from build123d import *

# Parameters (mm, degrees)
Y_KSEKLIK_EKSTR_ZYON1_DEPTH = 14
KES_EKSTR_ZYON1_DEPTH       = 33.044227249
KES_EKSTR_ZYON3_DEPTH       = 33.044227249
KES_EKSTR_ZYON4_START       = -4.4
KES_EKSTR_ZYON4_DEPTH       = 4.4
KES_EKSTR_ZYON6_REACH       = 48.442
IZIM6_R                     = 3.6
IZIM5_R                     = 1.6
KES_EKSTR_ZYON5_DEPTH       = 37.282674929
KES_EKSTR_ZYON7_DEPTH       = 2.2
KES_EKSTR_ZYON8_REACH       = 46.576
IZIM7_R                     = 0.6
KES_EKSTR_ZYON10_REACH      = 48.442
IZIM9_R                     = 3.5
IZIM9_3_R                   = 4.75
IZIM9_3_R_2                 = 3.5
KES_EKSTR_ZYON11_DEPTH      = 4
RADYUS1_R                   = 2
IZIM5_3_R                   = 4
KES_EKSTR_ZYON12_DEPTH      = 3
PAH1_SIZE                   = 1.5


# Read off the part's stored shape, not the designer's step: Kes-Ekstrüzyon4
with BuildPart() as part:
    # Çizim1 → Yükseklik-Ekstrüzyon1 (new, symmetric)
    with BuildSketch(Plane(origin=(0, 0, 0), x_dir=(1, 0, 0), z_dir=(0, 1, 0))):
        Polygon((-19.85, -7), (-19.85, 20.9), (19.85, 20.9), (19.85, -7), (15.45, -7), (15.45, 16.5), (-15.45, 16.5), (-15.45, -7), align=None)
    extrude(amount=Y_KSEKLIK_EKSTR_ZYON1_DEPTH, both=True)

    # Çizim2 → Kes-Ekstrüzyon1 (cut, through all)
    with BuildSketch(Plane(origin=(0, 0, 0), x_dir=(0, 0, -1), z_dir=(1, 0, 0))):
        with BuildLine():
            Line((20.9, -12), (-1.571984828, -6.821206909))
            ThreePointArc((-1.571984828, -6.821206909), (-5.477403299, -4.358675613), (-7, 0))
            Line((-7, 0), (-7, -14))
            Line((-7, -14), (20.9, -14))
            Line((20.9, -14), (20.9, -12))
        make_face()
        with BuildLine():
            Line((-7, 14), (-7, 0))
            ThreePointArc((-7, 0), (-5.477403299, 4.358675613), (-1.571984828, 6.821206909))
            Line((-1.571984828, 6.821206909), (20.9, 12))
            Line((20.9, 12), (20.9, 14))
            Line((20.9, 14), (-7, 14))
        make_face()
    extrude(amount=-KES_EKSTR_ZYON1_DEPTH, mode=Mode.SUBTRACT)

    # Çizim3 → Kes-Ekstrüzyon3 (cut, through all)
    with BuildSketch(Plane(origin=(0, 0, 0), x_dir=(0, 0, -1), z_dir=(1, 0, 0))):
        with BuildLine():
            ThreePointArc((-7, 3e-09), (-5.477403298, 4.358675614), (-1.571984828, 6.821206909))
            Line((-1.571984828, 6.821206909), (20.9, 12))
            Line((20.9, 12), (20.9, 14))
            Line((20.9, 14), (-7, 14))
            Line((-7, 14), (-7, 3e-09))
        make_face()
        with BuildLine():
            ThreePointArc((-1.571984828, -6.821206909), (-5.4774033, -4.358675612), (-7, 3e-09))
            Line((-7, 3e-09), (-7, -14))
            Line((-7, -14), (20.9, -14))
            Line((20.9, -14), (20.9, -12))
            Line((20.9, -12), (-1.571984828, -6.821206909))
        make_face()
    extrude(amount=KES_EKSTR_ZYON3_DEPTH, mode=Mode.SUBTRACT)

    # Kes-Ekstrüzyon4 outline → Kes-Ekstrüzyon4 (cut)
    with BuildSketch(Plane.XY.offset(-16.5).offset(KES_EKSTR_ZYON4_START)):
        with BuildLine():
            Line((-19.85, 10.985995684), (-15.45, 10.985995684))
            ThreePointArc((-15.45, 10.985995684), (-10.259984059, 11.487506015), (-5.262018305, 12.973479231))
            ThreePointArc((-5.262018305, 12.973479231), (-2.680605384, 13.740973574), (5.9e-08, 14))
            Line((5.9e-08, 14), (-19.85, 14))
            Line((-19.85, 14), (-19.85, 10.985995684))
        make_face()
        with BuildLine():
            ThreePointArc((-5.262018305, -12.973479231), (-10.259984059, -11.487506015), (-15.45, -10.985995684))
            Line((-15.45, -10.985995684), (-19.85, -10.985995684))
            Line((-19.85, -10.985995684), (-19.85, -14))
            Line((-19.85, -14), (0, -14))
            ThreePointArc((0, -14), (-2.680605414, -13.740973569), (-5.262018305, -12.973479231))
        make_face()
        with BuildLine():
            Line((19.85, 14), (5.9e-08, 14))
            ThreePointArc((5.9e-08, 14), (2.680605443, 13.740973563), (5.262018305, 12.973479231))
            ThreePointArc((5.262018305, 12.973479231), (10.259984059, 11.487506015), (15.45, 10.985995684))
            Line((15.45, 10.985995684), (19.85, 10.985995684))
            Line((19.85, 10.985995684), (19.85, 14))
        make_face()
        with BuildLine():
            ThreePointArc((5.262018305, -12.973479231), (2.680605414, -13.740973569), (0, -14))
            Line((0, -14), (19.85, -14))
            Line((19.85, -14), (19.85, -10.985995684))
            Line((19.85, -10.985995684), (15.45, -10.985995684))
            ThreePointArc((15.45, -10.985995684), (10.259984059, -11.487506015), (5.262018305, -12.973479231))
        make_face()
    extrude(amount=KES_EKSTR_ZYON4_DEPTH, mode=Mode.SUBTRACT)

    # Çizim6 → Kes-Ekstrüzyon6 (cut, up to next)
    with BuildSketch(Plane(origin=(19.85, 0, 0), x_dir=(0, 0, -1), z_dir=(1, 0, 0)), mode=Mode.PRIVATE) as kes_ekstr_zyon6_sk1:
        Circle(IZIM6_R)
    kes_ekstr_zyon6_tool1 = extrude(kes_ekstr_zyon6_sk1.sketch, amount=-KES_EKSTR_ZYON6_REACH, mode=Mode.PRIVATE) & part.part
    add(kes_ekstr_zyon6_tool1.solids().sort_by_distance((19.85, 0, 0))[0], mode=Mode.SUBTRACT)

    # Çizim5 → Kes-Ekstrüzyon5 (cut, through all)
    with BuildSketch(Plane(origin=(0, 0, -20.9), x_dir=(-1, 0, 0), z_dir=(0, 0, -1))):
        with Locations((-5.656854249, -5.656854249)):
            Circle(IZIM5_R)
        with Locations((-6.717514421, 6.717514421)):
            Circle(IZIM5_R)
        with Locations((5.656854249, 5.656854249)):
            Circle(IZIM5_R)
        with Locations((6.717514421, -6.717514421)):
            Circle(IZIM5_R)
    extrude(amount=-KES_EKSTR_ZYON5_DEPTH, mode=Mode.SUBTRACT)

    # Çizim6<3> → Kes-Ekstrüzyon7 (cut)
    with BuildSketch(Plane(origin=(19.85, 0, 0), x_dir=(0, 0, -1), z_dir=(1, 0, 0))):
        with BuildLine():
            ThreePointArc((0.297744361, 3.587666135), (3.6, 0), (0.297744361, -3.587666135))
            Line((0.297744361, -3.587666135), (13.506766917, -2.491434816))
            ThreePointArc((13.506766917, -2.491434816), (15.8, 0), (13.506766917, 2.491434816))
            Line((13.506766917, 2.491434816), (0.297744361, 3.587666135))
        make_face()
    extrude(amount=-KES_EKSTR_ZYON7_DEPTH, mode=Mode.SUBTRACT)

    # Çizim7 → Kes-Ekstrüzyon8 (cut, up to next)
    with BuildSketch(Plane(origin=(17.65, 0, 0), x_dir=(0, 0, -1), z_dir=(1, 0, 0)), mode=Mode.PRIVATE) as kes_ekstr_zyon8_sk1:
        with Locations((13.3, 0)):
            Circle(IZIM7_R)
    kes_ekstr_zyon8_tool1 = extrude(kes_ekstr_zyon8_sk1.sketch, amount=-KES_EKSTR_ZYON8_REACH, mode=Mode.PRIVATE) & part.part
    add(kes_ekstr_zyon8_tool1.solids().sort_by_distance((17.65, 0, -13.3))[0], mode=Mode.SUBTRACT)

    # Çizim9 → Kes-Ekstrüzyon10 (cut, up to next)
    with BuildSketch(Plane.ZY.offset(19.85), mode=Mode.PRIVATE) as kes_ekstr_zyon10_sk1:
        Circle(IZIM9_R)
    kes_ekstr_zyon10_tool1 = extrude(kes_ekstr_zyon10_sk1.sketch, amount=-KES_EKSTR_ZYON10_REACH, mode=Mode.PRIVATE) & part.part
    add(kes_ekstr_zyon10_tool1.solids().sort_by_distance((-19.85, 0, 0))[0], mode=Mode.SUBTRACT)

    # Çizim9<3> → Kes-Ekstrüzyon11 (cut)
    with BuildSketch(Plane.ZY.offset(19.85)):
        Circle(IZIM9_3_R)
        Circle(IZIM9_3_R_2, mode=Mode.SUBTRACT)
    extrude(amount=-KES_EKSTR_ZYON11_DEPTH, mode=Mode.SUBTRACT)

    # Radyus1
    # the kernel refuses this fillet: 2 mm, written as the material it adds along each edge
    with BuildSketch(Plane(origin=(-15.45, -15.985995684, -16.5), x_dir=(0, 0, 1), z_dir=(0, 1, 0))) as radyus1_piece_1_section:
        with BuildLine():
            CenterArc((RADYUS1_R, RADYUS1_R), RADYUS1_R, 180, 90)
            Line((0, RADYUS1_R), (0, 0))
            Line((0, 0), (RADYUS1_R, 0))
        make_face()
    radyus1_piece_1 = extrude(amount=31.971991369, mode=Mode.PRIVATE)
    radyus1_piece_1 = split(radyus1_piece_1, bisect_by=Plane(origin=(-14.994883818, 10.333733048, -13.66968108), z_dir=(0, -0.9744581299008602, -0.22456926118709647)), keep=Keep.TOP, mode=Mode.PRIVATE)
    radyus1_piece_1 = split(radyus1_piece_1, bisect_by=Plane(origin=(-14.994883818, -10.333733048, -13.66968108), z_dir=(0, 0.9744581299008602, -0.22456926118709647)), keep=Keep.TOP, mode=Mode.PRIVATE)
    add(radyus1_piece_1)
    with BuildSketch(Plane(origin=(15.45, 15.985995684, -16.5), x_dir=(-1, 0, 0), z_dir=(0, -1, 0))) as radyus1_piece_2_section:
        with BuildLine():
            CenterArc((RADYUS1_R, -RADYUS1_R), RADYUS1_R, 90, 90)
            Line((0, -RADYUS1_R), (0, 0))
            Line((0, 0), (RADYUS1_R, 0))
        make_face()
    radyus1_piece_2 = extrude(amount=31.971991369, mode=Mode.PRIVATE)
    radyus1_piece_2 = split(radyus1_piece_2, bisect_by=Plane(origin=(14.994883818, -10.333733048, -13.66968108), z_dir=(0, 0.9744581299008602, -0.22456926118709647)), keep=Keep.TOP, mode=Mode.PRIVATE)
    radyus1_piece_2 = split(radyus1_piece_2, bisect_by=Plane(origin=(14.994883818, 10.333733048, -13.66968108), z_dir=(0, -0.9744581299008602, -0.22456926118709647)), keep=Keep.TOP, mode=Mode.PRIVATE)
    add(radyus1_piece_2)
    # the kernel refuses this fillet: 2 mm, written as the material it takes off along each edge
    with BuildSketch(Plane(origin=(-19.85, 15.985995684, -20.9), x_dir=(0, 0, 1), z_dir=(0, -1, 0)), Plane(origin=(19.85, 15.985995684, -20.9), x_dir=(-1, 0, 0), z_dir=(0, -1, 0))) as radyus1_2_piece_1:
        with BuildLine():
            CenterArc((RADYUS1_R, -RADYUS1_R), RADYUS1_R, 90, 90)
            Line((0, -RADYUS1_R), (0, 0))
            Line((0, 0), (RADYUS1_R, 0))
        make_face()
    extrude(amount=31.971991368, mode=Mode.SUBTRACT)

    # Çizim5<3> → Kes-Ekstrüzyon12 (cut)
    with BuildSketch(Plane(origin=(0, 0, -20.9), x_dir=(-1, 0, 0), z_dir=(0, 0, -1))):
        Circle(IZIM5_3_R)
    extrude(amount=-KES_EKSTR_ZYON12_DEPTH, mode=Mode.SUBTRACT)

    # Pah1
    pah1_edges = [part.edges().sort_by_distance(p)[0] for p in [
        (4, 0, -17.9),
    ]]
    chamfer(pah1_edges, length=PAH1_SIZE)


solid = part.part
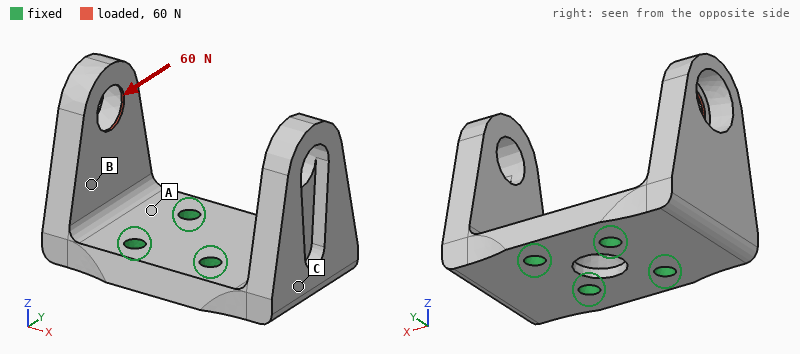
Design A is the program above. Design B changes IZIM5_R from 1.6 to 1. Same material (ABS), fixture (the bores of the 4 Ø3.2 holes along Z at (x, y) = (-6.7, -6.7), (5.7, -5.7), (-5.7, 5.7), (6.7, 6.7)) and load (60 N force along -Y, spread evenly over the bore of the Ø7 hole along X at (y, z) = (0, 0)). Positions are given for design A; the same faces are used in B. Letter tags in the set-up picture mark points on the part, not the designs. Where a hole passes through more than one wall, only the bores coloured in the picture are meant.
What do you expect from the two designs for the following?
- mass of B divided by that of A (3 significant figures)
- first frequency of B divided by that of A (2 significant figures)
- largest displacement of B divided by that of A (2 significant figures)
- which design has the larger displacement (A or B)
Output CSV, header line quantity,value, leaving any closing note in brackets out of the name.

quantity,value
mass of B divided by that of A,1.01
first frequency of B divided by that of A,0.96
largest displacement of B divided by that of A,1.1
which design has the larger displacement,B
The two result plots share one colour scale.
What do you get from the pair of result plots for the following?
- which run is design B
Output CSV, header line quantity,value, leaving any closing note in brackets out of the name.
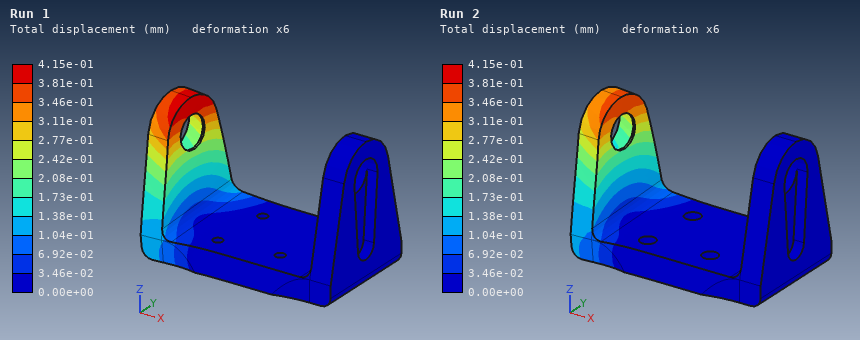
quantity,value
which run is design B,Run 1
